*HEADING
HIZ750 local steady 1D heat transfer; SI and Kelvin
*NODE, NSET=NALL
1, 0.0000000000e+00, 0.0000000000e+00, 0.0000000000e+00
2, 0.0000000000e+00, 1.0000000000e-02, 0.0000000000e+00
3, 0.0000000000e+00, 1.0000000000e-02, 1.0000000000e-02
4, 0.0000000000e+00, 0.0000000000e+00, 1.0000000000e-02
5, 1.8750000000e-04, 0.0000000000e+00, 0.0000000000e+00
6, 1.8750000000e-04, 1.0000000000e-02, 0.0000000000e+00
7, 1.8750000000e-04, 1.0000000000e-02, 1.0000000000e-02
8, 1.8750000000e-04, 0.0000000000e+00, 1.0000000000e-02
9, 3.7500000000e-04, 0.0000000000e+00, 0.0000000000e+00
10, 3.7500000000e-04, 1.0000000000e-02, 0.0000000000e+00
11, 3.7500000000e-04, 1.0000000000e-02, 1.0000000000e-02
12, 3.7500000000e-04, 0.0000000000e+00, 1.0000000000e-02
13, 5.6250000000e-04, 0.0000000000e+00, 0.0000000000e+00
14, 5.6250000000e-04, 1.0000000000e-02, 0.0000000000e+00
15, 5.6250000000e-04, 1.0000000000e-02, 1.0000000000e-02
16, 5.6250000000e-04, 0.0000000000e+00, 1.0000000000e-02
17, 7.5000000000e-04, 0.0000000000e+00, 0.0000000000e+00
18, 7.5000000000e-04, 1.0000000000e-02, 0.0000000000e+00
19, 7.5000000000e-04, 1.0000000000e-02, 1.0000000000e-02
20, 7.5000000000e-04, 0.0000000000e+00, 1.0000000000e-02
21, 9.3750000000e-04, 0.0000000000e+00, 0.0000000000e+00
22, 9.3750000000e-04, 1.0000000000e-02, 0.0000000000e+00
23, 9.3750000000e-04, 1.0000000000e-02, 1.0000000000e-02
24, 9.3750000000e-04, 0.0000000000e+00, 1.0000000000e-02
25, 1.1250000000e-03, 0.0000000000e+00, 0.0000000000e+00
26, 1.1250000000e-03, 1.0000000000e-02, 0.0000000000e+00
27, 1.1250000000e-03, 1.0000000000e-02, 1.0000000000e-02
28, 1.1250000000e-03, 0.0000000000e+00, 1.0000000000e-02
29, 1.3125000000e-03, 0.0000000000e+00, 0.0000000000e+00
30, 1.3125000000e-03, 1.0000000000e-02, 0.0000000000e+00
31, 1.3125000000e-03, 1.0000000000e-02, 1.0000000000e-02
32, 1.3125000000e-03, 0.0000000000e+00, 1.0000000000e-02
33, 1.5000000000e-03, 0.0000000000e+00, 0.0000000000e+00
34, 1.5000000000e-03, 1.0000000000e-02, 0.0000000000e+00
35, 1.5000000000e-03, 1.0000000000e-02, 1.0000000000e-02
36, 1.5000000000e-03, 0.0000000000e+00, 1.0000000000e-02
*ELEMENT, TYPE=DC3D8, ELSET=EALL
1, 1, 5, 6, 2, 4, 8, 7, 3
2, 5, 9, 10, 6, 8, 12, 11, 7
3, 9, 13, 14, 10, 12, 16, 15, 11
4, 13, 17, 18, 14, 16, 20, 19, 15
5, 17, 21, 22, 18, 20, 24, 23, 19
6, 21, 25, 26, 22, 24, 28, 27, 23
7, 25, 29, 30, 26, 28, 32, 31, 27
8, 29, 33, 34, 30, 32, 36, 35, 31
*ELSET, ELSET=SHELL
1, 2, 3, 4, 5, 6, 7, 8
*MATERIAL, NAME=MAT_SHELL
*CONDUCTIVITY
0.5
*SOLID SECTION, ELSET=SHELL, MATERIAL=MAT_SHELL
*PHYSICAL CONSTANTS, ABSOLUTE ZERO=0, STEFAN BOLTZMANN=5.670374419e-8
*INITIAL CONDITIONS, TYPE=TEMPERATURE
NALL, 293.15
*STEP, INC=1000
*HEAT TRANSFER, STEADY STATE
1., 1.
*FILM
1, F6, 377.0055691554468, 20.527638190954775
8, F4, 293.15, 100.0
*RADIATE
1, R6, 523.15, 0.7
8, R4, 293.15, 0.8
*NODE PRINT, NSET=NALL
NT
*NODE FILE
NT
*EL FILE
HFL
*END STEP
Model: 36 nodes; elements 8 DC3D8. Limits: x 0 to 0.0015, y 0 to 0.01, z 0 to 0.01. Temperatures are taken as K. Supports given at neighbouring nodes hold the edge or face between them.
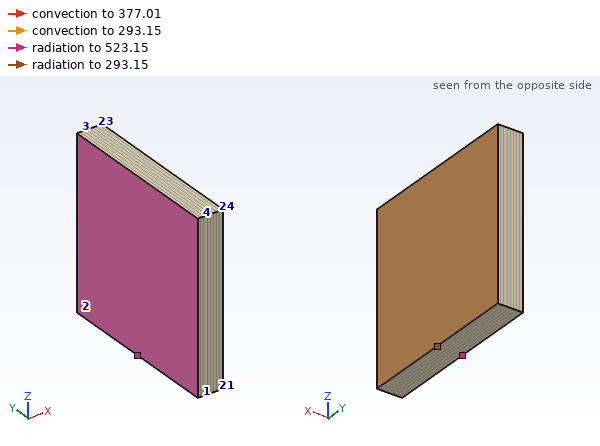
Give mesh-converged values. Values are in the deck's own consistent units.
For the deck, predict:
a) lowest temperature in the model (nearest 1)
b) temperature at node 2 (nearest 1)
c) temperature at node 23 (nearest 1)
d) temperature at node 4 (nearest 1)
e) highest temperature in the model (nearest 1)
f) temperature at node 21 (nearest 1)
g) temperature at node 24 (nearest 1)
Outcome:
325 K
335 K
329 K
335 K
335 K
329 K
329 K
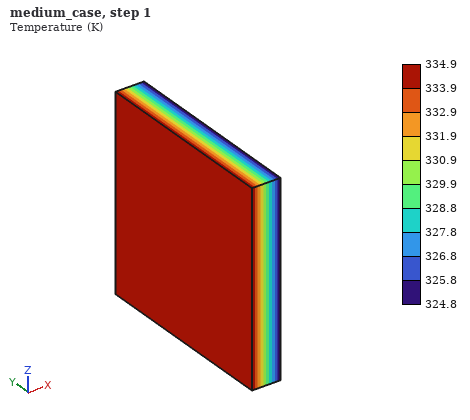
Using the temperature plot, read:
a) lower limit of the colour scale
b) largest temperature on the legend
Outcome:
324.8 K
334.9 K
